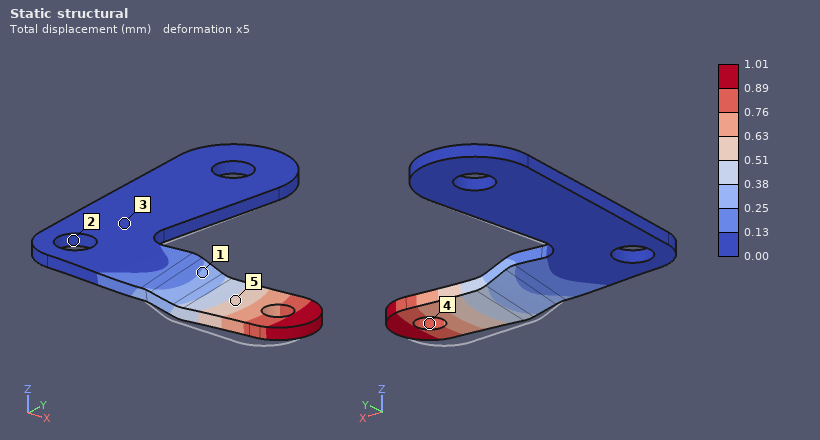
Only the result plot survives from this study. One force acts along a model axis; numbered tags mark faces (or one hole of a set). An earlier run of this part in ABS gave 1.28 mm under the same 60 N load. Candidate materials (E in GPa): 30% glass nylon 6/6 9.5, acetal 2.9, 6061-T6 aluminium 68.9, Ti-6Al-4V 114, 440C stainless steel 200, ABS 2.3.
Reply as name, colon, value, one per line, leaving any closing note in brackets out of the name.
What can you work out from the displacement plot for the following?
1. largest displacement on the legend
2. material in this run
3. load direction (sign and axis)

largest displacement on the legend: 1.01 mm
material in this run: acetal
load direction: +Y
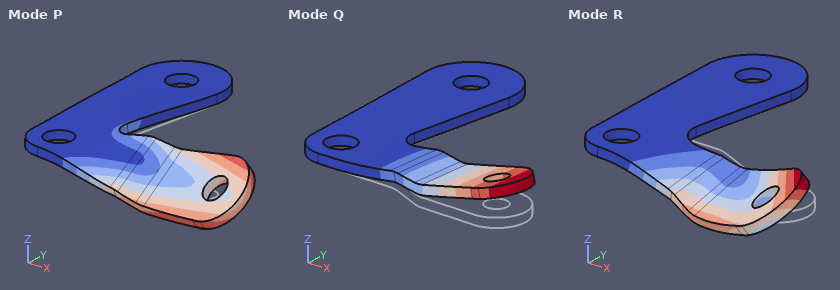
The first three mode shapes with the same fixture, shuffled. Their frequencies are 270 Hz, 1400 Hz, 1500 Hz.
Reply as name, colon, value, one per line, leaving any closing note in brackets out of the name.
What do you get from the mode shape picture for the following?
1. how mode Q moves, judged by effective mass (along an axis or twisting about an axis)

how mode Q moves, judged by effective mass: along Z
